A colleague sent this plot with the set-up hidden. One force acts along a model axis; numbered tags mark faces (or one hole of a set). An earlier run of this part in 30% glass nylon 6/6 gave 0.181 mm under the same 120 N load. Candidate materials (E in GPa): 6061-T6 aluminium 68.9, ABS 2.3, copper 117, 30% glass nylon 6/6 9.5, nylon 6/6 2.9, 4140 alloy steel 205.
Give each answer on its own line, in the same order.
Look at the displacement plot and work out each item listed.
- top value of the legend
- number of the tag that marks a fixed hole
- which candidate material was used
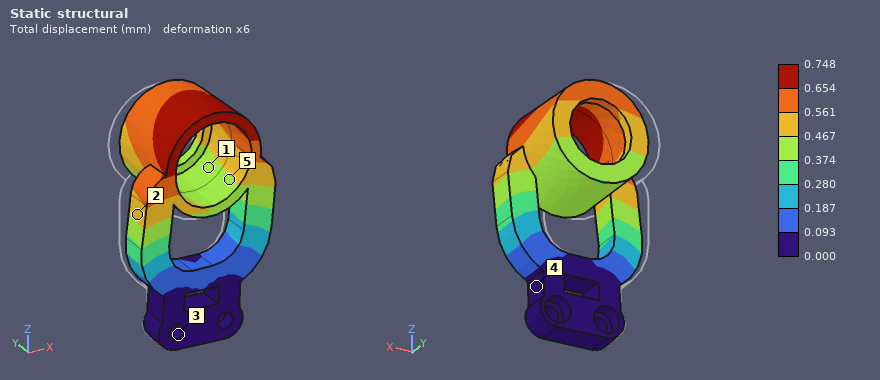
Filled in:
0.748 mm
3
ABS
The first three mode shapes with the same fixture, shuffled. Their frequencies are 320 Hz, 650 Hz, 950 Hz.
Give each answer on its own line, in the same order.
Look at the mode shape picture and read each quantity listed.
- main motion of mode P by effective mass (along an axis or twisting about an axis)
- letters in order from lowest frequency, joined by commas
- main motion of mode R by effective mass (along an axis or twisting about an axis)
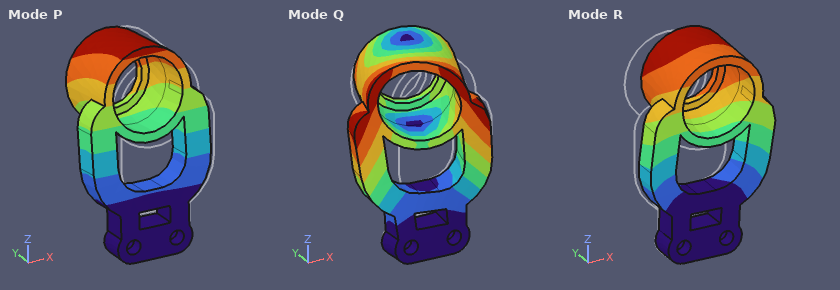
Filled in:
along Y
P, R, Q
along X
